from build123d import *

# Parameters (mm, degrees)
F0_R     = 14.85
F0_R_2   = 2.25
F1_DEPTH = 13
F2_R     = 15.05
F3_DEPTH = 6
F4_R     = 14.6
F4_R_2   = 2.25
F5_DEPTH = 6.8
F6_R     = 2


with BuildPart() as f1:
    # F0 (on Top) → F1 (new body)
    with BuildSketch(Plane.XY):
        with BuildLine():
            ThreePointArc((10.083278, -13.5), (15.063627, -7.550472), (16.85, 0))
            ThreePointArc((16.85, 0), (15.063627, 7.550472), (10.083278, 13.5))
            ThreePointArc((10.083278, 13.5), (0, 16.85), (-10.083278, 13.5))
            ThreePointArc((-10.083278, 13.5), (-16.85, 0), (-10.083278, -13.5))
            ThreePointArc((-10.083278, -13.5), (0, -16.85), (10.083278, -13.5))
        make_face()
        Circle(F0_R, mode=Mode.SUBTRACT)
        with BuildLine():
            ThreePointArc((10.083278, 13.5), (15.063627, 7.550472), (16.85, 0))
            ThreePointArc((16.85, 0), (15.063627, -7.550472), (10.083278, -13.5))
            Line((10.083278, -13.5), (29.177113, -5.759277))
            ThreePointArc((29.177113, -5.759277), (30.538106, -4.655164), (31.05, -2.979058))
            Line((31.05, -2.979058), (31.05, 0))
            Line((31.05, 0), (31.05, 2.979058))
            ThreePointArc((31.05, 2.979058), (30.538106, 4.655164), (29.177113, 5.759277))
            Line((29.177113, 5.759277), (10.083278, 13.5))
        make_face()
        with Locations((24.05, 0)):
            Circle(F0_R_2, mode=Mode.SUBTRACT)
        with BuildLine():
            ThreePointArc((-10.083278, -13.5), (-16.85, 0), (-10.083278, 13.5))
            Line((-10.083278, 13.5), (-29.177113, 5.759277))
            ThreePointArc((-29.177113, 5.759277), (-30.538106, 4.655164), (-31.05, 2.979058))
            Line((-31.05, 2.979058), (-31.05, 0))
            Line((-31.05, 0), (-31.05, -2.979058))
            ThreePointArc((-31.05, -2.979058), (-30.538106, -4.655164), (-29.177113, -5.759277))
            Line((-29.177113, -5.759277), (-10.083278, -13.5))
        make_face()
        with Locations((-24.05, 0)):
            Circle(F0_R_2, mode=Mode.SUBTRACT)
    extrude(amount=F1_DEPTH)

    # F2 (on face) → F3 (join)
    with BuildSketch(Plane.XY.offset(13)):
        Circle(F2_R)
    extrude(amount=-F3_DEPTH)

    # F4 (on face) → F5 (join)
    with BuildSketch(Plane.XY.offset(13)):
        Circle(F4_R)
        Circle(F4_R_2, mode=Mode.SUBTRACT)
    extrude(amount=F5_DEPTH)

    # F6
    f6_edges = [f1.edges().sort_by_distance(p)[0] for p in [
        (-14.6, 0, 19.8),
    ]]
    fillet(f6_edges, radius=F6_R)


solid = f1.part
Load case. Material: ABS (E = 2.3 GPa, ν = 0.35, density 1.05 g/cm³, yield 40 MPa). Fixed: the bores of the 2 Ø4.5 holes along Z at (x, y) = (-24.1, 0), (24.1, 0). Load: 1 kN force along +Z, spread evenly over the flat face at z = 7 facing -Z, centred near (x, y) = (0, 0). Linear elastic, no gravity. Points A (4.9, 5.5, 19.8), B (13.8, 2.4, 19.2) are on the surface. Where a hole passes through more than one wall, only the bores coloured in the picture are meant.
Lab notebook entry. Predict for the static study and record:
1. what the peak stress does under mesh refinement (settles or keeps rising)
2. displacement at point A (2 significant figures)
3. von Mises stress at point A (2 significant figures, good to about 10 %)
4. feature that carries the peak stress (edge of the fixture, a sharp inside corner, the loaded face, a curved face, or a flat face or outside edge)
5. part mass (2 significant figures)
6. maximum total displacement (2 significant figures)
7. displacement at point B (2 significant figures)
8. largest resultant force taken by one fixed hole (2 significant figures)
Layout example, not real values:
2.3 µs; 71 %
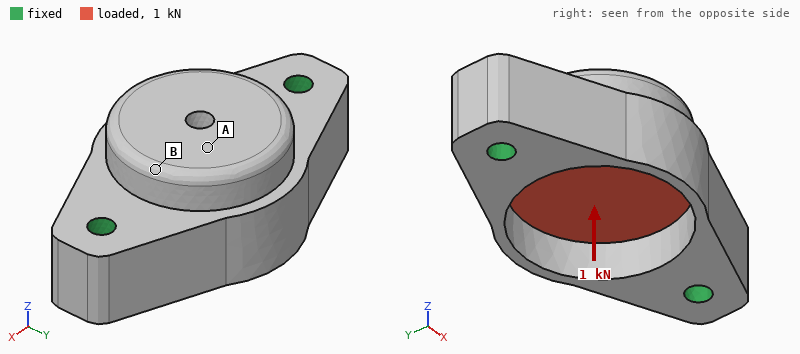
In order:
keeps rising; 0.085 mm; 4.3 MPa; edge of the fixture; 18 g; 0.12 mm; 0.065 mm; 590 N
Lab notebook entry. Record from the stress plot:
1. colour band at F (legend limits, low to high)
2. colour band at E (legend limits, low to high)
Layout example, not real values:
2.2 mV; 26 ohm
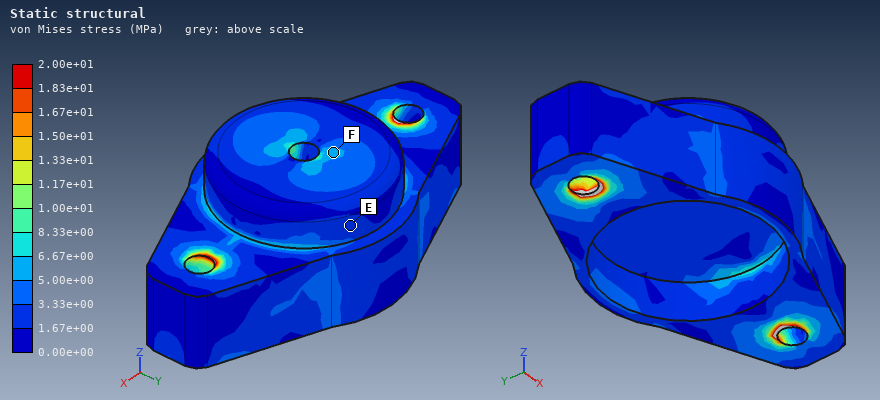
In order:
5.00e+00 to 6.67e+00 MPa; 1.67e+00 to 3.33e+00 MPa
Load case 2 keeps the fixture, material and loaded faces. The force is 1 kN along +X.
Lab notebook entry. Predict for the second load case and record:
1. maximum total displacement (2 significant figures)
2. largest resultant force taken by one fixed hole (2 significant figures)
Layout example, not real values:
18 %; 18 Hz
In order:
37 µm; 500 N
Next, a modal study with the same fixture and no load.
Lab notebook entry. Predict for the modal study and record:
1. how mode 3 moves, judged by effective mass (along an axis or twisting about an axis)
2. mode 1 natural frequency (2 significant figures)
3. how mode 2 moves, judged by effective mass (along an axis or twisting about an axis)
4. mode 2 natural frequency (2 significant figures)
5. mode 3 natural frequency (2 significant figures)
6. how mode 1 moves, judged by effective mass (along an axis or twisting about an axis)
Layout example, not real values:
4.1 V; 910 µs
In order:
along Y; 3700 Hz; along Z; 5000 Hz; 6800 Hz; along Y
